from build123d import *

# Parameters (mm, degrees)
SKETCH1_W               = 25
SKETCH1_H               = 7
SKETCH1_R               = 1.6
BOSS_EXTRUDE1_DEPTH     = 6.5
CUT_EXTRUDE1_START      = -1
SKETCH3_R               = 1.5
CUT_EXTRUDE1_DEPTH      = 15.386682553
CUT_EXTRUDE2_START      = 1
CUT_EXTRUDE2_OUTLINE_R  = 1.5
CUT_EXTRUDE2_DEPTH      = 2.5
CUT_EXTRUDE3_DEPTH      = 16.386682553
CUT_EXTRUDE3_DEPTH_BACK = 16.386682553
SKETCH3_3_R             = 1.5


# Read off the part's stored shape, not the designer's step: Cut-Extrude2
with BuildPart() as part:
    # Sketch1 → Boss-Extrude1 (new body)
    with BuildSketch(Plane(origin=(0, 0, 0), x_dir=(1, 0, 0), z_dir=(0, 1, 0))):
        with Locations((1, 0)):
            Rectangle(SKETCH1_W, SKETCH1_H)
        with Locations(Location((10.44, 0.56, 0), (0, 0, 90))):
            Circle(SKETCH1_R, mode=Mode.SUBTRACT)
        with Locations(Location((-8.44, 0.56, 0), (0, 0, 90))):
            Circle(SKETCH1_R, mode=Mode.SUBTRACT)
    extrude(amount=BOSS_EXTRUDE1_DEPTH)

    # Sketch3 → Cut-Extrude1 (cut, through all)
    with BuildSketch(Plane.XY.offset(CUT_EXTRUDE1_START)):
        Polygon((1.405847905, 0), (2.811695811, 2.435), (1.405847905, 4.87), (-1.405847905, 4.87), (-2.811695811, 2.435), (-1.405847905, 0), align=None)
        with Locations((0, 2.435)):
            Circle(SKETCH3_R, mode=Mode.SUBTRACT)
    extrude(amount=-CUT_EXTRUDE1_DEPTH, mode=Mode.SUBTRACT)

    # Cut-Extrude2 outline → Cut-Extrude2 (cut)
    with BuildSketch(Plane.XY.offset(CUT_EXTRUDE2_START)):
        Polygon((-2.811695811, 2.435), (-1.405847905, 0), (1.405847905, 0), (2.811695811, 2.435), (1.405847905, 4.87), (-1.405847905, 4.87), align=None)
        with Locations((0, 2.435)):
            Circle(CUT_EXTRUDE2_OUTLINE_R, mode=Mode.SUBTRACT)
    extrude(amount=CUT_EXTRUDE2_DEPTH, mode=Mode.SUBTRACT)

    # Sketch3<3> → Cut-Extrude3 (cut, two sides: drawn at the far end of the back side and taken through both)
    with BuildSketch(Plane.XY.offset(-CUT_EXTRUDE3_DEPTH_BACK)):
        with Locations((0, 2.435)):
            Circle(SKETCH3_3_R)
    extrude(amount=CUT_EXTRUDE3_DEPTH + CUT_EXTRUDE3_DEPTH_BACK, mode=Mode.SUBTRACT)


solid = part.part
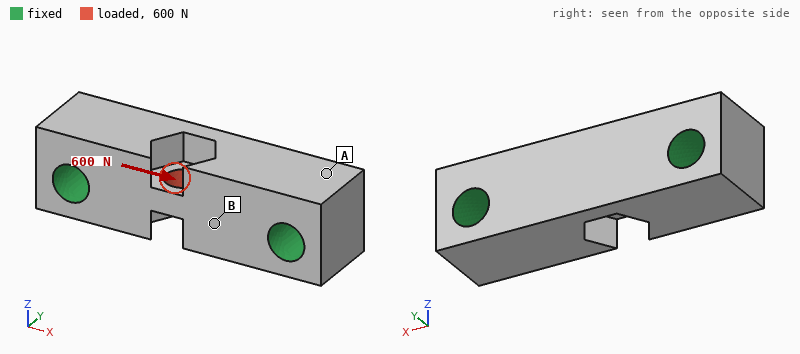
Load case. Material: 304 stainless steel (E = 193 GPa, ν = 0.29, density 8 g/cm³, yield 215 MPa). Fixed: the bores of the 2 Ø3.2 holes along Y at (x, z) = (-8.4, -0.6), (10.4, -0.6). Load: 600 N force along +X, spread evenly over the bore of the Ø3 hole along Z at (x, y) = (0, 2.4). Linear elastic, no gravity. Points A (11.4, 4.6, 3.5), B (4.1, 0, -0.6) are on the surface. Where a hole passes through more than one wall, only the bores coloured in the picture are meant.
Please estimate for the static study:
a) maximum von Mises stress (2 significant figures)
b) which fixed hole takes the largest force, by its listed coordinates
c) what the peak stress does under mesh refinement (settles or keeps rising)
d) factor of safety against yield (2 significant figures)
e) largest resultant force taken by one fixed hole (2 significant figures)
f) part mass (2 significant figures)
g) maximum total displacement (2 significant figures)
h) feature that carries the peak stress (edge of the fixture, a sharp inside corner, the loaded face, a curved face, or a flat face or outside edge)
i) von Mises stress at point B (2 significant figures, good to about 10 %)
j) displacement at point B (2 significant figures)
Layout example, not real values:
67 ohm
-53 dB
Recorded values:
60 MPa
(-8.4, -0.6)
settles
3.6
320 N
7.3 g
0.81 µm
the loaded face
18 MPa
0.31 µm
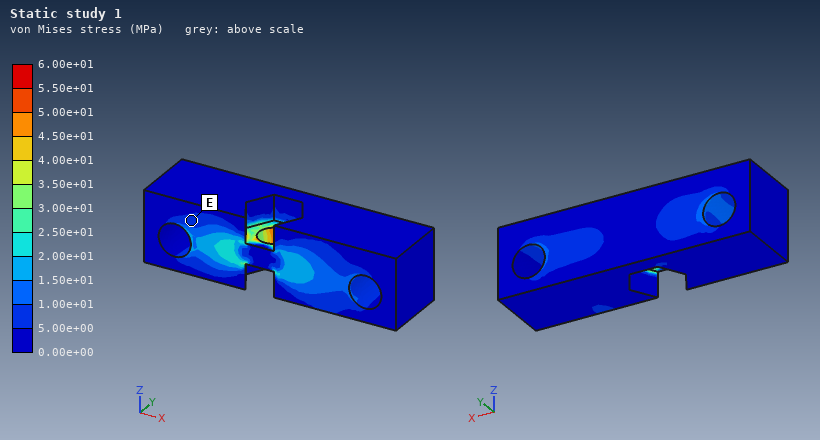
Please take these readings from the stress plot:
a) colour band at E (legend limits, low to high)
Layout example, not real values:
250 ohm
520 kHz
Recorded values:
5.00e+00 to 1.00e+01 MPa
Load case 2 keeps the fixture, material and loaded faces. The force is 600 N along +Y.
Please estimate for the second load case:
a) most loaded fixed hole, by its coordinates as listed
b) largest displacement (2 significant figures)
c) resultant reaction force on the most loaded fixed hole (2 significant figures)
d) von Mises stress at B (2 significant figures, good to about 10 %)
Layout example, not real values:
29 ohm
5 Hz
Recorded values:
(-8.4, -0.6)
2.8 µm
340 N
12 MPa
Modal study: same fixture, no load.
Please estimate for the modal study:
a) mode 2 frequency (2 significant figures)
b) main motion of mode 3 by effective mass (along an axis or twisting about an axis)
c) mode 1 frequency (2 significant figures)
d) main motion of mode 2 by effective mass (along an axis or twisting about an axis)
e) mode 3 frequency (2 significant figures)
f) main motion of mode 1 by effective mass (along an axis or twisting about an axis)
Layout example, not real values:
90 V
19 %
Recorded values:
70 kHz
twisting about X
61 kHz
along Y
88 kHz
along Z
